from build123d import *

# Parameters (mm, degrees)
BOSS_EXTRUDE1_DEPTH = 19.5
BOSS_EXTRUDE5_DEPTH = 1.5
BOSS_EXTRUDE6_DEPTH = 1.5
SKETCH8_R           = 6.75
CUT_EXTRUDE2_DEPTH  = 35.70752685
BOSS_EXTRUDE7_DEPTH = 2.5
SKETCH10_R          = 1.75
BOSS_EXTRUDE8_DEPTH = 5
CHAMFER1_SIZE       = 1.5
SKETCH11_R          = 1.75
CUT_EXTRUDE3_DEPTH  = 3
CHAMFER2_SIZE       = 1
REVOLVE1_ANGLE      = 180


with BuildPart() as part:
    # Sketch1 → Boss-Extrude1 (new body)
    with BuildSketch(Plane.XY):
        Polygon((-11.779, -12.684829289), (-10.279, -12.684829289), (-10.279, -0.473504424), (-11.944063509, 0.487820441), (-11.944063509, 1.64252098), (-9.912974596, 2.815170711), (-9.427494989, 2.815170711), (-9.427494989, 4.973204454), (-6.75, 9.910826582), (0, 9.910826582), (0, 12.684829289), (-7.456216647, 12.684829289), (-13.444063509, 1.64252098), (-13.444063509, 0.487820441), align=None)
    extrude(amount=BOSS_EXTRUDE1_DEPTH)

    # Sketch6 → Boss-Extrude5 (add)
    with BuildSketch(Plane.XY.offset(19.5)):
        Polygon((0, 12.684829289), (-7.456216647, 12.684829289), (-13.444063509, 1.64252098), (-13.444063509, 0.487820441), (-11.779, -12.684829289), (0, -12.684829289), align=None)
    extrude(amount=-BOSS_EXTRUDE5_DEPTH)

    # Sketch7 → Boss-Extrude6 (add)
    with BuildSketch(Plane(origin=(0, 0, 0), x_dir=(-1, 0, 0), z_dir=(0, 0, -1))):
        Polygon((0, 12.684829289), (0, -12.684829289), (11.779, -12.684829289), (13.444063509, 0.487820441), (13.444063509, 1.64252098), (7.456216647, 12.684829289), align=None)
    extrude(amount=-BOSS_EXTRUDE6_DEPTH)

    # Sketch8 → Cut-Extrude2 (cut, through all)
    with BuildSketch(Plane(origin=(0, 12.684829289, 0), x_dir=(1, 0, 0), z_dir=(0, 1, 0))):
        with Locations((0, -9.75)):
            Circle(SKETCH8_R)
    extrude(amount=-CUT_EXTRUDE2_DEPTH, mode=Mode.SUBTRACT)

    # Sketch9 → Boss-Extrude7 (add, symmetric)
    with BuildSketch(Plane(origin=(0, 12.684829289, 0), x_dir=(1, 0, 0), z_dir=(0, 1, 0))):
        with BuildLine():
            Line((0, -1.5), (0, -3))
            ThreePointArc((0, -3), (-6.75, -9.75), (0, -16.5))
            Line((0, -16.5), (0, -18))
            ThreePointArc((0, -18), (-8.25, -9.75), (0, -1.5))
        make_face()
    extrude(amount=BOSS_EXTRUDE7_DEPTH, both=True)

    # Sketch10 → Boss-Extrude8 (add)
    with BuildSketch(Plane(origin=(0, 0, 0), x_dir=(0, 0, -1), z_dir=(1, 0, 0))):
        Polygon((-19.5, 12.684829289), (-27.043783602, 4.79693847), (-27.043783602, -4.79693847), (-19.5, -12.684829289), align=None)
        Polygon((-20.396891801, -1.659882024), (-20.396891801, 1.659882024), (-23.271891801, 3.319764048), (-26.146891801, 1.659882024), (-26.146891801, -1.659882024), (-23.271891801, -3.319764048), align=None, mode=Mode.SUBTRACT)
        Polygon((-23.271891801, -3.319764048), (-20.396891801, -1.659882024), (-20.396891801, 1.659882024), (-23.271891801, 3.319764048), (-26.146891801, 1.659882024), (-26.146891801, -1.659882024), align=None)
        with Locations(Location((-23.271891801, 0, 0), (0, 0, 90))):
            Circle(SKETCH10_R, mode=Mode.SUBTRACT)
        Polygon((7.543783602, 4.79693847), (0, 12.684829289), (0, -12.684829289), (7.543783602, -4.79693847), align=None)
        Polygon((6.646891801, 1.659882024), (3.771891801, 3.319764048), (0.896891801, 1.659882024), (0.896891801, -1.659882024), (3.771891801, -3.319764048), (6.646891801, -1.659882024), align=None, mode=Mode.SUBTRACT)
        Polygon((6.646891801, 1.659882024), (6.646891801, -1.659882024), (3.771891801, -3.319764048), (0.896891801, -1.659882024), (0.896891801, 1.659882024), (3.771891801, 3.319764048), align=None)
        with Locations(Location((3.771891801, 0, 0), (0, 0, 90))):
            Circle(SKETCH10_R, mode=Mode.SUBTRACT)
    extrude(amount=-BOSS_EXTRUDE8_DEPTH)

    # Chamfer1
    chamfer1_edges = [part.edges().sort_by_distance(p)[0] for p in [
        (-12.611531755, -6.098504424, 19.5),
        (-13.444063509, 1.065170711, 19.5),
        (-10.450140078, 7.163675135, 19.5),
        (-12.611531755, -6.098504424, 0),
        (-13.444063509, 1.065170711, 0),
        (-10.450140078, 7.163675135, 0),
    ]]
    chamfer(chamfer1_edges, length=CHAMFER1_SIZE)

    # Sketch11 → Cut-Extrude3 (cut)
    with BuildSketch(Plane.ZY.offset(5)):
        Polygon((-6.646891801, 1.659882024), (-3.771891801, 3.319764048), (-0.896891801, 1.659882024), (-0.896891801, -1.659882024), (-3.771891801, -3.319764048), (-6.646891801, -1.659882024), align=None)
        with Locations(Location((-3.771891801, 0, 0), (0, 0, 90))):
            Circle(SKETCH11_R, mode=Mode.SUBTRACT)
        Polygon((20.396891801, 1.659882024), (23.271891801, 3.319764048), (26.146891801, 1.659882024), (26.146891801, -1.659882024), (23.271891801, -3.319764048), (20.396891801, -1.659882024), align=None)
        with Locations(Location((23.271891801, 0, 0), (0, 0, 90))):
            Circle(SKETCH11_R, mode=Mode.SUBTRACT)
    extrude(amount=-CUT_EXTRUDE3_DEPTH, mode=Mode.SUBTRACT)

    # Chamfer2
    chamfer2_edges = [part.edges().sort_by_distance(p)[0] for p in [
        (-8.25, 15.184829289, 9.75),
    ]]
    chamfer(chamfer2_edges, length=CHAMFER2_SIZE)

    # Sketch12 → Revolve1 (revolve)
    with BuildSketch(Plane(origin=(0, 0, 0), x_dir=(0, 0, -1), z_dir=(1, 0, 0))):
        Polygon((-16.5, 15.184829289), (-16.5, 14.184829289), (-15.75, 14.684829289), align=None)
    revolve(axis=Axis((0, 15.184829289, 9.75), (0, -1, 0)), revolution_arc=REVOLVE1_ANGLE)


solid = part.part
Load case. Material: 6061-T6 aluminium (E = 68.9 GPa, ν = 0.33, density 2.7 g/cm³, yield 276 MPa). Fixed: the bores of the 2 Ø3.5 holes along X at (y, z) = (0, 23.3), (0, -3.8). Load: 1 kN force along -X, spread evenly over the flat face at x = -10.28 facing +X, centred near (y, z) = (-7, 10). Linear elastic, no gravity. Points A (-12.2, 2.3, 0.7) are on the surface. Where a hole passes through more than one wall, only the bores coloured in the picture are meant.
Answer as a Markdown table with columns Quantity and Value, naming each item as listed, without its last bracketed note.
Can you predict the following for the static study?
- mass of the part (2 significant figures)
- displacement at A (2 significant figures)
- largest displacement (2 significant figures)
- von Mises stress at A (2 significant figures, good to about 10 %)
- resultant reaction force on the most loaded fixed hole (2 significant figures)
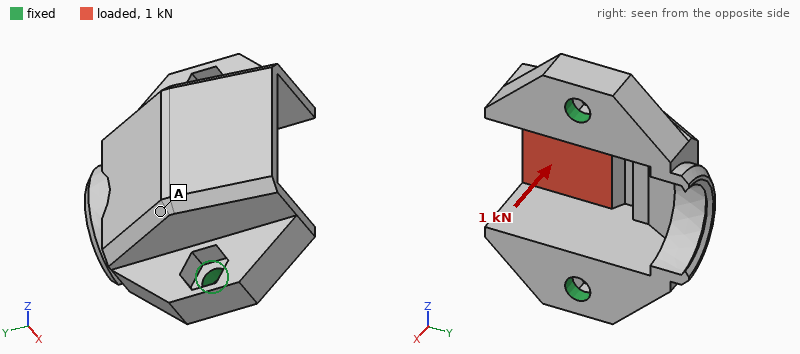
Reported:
| Quantity | Value |
|---|---|
| mass of the part | 8.2 g |
| displacement at A | 0.049 mm |
| largest displacement | 0.13 mm |
| von Mises stress at A | 28 MPa |
| resultant reaction force on the most loaded fixed hole | 570 N |
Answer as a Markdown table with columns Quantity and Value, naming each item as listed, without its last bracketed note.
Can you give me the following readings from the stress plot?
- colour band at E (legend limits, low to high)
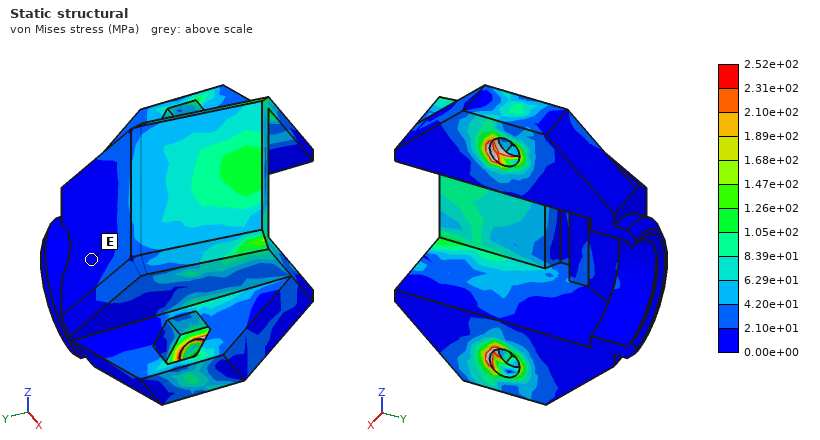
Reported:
| Quantity | Value |
|---|---|
| colour band at E | 0.00e+00 to 2.10e+01 MPa |
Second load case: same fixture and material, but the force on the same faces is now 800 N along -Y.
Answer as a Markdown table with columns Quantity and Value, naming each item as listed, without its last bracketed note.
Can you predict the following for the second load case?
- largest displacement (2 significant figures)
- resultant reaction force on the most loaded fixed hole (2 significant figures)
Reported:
| Quantity | Value |
|---|---|
| largest displacement | 89 µm |
| resultant reaction force on the most loaded fixed hole | 400 N |
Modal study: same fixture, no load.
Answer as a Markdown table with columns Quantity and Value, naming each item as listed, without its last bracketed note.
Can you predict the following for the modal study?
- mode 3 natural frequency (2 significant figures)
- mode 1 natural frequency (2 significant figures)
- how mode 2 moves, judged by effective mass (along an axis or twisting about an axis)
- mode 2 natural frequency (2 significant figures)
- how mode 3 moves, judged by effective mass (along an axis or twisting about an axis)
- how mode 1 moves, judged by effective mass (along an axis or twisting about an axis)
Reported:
| Quantity | Value |
|---|---|
| mode 3 natural frequency | 16 kHz |
| mode 1 natural frequency | 7200 Hz |
| how mode 2 moves, judged by effective mass | along Z |
| mode 2 natural frequency | 12 kHz |
| how mode 3 moves, judged by effective mass | along Z |
| how mode 1 moves, judged by effective mass | along Y |
